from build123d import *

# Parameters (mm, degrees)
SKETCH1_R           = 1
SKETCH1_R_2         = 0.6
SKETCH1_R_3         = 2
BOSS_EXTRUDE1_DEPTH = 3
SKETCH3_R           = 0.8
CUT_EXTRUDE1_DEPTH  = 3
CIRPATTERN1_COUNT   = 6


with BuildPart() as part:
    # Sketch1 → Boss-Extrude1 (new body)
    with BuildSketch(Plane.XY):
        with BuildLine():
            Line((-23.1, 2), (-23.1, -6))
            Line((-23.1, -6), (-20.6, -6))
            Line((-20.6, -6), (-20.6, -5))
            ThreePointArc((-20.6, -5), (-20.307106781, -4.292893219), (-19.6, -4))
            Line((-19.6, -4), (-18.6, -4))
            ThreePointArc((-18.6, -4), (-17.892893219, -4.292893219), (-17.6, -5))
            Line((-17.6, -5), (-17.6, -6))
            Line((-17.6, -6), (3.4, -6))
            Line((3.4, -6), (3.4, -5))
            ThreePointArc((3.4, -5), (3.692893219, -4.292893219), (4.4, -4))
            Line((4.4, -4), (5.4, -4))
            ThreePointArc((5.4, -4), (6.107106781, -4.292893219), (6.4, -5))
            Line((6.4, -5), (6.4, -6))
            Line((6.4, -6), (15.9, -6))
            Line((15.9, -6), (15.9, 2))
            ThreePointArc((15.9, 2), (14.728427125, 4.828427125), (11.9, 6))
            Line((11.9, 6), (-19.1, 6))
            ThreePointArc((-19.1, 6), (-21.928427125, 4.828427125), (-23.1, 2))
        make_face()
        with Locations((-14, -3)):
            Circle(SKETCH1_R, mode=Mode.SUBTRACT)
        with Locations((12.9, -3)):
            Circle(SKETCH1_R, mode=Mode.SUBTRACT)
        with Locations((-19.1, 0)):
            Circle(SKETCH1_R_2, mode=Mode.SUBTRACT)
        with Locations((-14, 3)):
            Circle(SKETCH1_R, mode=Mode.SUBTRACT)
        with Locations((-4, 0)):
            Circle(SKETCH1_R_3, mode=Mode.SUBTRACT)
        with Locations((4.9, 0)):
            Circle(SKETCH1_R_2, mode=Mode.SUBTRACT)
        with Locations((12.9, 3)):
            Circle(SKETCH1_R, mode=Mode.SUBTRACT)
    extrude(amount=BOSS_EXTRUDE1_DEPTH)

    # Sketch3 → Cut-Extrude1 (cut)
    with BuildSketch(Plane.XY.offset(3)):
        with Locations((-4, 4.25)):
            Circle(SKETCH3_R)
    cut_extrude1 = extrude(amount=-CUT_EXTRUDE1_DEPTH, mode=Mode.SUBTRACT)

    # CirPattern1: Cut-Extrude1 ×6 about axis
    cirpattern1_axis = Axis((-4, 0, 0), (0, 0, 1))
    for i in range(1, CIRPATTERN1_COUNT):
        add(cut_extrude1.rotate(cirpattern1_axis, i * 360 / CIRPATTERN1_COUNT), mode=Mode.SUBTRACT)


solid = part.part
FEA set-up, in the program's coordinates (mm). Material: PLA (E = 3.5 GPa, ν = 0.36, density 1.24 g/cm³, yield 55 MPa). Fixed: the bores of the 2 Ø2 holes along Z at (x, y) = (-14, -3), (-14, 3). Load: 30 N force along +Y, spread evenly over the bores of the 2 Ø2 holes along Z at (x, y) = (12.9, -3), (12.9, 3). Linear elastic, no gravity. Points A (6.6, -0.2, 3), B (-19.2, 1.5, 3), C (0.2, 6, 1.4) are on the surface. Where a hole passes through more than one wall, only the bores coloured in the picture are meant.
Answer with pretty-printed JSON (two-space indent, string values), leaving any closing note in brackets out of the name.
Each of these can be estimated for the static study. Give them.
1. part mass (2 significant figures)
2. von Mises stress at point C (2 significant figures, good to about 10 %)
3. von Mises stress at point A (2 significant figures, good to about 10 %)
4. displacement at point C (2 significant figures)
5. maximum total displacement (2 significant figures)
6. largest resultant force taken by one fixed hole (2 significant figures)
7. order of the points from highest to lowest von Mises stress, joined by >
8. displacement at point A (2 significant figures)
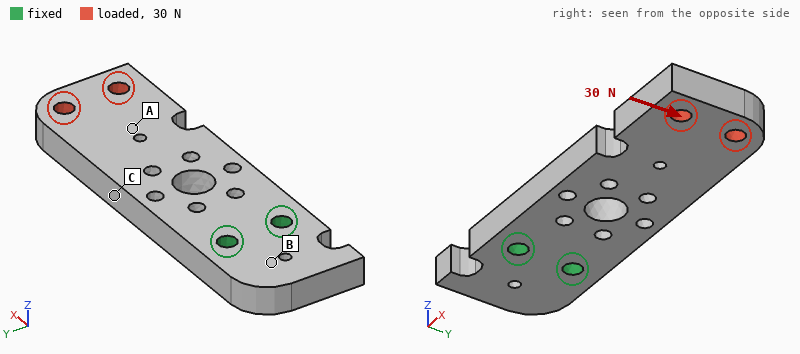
{
  "part mass": "1.5 g",
  "von Mises stress at point C": "5.3 MPa",
  "von Mises stress at point A": "3.3 MPa",
  "displacement at point C": "0.087 mm",
  "maximum total displacement": "0.23 mm",
  "largest resultant force taken by one fixed hole": "110 N",
  "order of the points from highest to lowest von Mises stress, joined by >": "C > A > B",
  "displacement at point A": "0.13 mm"
}
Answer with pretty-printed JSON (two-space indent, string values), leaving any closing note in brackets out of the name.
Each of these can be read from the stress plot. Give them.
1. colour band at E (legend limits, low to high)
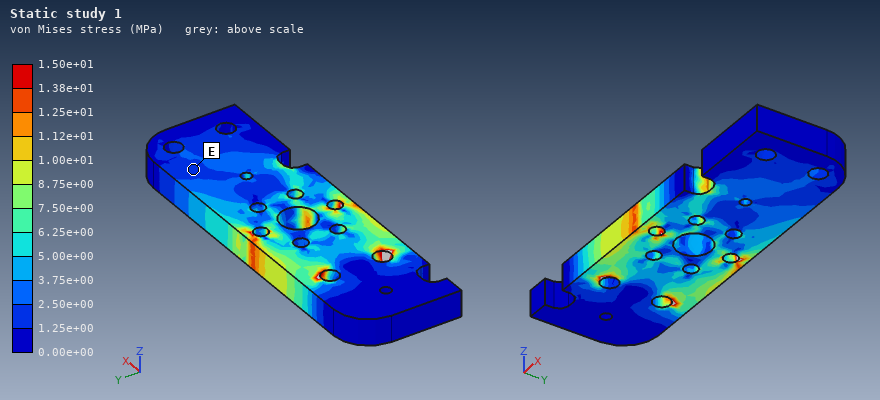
{
  "colour band at E": "1.25e+00 to 2.50e+00 MPa"
}
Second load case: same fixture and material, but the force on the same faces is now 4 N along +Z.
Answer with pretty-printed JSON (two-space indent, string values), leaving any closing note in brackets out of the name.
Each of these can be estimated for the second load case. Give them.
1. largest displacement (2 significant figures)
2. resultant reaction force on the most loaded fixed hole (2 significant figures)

{
  "largest displacement": "0.41 mm",
  "resultant reaction force on the most loaded fixed hole": "2.0 N"
}
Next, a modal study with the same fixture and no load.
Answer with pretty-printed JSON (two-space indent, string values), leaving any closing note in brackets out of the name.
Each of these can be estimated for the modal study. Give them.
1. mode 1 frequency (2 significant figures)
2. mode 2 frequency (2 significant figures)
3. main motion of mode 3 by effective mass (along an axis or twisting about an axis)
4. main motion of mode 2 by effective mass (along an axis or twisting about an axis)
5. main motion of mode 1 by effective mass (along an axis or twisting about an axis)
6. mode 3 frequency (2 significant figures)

{
  "mode 1 frequency": "870 Hz",
  "mode 2 frequency": "3000 Hz",
  "main motion of mode 3 by effective mass": "twisting about X",
  "main motion of mode 2 by effective mass": "along Y",
  "main motion of mode 1 by effective mass": "along Z",
  "mode 3 frequency": "3800 Hz"
}
